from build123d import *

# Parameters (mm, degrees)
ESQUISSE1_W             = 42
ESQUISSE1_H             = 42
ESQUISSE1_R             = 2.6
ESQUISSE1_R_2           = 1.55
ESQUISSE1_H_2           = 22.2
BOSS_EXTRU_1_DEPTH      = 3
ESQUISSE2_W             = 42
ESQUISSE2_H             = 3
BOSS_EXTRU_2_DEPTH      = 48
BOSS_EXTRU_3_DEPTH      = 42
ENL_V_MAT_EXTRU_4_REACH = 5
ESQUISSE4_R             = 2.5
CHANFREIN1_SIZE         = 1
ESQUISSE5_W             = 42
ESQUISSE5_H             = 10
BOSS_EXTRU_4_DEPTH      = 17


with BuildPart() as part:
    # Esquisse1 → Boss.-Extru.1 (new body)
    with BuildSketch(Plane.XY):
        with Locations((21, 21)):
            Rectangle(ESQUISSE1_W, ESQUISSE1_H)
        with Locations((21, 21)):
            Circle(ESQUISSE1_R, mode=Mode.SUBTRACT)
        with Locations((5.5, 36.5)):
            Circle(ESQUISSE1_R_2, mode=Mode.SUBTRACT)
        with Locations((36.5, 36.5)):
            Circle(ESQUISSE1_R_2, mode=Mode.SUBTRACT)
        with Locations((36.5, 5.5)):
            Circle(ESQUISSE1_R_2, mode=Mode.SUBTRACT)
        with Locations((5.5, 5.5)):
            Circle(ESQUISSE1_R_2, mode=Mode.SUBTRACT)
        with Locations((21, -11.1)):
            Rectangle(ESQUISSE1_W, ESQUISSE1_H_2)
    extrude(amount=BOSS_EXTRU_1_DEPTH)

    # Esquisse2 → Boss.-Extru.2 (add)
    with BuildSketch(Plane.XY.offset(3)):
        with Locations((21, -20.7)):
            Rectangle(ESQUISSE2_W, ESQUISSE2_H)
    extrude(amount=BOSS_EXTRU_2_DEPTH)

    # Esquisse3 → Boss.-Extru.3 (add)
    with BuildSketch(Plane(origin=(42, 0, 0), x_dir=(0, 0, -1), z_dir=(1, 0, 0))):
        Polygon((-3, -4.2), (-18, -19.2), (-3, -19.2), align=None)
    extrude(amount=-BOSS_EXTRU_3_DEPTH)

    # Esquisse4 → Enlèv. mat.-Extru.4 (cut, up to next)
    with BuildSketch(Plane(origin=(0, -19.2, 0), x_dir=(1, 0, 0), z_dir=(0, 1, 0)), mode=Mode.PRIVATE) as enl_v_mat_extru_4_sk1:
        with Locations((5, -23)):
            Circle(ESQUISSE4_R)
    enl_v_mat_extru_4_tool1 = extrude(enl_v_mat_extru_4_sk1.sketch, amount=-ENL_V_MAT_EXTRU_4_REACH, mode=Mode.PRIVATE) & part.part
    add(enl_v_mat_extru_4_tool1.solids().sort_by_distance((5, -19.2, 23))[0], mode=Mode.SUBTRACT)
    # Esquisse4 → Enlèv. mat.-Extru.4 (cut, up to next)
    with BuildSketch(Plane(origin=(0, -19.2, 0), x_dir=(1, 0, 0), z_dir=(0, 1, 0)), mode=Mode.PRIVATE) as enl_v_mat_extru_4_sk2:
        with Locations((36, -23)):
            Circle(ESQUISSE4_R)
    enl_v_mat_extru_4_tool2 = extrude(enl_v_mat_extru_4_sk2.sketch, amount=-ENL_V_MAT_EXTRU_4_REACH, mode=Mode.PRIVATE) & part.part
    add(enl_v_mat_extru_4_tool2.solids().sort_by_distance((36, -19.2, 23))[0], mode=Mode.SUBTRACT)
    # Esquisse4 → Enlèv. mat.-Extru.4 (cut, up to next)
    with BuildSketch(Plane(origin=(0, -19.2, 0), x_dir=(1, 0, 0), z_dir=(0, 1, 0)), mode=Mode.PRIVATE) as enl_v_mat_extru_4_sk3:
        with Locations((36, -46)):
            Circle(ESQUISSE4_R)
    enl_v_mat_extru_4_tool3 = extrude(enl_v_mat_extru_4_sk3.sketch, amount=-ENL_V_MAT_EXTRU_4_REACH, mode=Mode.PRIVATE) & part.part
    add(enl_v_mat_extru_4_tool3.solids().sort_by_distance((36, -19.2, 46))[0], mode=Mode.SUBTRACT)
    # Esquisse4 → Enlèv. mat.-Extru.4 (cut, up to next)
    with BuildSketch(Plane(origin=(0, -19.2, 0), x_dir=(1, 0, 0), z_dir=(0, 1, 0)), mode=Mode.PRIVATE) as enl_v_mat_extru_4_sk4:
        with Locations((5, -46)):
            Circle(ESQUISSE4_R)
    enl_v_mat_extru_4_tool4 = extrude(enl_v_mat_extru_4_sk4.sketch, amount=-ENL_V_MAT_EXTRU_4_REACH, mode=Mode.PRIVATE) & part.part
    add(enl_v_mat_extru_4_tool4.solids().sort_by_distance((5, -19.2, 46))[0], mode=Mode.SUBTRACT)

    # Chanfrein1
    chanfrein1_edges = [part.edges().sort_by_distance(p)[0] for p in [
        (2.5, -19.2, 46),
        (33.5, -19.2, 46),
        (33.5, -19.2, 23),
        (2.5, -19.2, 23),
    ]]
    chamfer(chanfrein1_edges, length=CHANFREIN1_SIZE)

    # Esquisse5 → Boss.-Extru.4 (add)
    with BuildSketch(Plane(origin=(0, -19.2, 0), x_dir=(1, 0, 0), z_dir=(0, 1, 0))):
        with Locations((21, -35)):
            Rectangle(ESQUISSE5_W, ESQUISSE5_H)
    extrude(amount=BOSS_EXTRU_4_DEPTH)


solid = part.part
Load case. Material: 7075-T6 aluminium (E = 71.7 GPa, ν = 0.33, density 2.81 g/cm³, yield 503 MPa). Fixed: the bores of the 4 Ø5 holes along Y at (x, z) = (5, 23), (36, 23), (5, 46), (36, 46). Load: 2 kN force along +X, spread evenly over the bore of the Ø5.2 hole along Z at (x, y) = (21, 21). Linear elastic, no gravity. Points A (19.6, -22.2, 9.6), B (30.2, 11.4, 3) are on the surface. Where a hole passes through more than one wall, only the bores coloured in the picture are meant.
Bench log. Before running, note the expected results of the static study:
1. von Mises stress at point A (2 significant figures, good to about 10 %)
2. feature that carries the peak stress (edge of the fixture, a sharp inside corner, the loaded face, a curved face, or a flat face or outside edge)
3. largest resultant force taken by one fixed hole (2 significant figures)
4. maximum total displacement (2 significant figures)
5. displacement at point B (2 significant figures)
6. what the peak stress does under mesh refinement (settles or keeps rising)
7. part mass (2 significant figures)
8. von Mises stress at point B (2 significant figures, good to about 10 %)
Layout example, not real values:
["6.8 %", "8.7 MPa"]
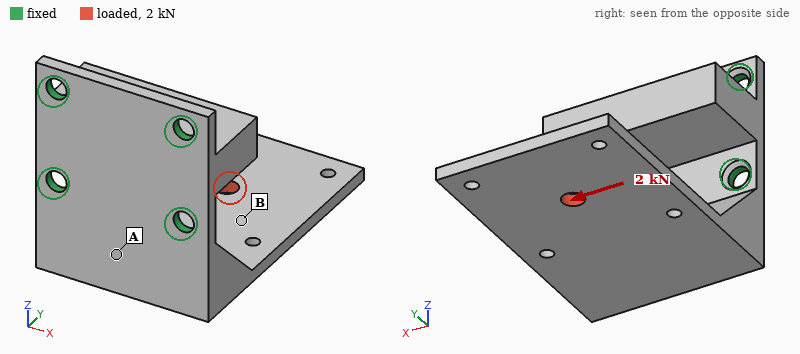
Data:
["100 MPa", "edge of the fixture", "3.2 kN", "0.54 mm", "0.26 mm", "keeps rising", "72 g", "41 MPa"]
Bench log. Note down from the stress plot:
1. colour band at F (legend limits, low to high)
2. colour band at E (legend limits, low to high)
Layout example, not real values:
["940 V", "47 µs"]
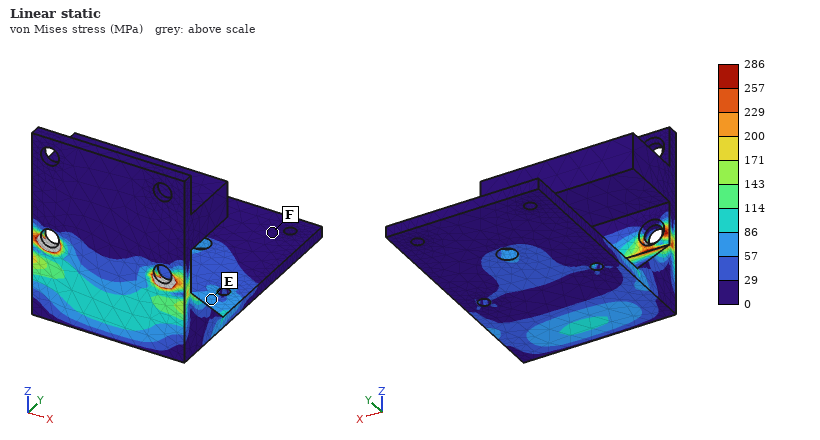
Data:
["0 to 29 MPa", "57 to 86 MPa"]
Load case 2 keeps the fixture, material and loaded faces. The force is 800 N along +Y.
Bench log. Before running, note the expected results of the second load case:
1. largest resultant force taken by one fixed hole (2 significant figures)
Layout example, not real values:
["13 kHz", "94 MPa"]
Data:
["590 N"]
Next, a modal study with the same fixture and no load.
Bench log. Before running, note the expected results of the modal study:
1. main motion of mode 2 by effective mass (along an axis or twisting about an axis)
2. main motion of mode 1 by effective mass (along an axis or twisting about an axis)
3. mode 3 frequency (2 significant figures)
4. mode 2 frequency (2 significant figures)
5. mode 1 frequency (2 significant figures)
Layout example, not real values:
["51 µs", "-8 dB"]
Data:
["along Y", "along Z", "2600 Hz", "2100 Hz", "670 Hz"]
